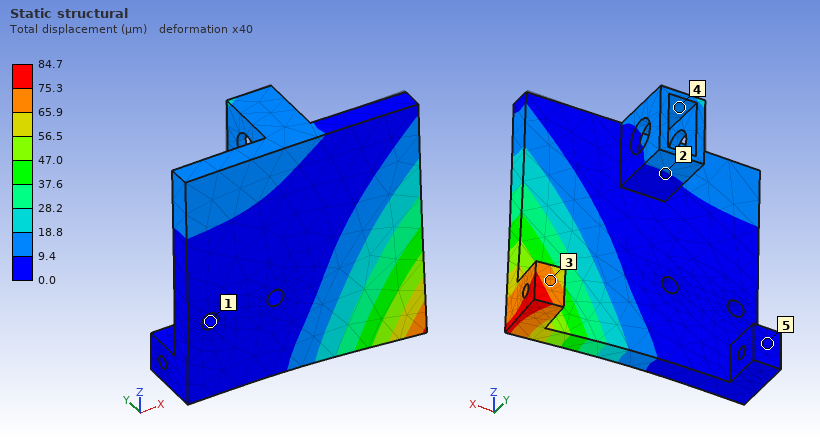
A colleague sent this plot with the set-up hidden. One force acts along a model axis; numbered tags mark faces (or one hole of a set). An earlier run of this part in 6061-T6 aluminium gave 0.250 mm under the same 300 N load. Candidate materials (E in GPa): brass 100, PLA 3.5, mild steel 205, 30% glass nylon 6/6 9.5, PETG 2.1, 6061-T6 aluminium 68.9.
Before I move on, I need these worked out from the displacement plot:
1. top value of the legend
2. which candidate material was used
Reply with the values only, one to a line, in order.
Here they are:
84.7 µm
mild steel
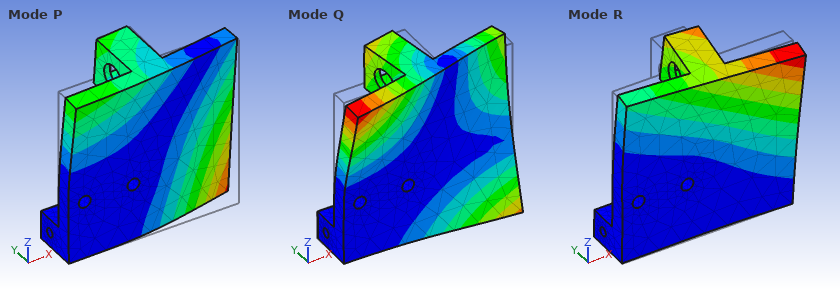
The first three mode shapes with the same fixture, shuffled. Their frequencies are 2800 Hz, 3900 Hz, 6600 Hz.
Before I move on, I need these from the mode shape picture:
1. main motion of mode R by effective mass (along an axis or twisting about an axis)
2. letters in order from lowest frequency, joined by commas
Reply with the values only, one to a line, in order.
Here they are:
along Y
R, P, Q
